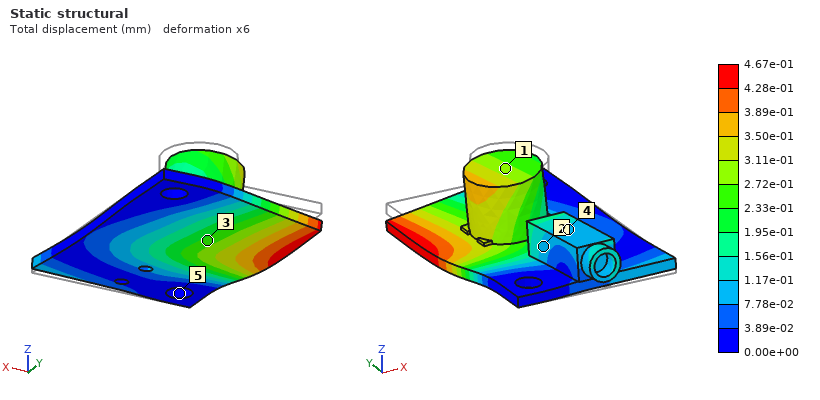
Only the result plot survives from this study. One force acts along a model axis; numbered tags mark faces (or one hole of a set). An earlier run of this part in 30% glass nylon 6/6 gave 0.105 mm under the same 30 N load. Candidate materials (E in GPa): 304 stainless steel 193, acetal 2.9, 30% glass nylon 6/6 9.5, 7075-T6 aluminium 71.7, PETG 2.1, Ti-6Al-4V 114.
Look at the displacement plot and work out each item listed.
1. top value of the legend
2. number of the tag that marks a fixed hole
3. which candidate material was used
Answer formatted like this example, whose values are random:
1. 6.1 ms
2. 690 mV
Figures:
1. 4.67e-01 mm
2. 5
3. PETG
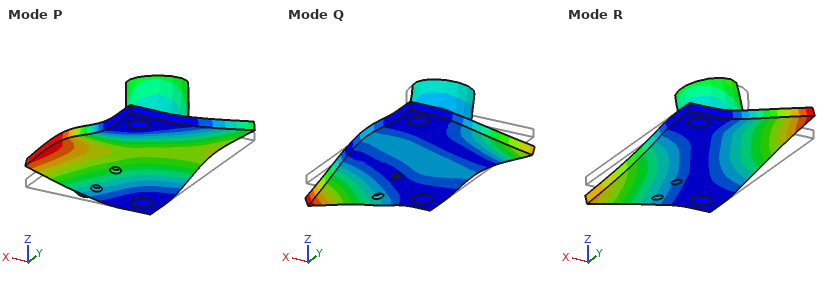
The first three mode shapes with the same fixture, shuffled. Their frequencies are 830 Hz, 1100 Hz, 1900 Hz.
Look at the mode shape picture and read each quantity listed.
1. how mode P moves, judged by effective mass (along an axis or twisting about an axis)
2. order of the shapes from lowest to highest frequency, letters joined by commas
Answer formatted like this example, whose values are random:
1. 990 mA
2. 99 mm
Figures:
1. along Z
2. R, P, Q
